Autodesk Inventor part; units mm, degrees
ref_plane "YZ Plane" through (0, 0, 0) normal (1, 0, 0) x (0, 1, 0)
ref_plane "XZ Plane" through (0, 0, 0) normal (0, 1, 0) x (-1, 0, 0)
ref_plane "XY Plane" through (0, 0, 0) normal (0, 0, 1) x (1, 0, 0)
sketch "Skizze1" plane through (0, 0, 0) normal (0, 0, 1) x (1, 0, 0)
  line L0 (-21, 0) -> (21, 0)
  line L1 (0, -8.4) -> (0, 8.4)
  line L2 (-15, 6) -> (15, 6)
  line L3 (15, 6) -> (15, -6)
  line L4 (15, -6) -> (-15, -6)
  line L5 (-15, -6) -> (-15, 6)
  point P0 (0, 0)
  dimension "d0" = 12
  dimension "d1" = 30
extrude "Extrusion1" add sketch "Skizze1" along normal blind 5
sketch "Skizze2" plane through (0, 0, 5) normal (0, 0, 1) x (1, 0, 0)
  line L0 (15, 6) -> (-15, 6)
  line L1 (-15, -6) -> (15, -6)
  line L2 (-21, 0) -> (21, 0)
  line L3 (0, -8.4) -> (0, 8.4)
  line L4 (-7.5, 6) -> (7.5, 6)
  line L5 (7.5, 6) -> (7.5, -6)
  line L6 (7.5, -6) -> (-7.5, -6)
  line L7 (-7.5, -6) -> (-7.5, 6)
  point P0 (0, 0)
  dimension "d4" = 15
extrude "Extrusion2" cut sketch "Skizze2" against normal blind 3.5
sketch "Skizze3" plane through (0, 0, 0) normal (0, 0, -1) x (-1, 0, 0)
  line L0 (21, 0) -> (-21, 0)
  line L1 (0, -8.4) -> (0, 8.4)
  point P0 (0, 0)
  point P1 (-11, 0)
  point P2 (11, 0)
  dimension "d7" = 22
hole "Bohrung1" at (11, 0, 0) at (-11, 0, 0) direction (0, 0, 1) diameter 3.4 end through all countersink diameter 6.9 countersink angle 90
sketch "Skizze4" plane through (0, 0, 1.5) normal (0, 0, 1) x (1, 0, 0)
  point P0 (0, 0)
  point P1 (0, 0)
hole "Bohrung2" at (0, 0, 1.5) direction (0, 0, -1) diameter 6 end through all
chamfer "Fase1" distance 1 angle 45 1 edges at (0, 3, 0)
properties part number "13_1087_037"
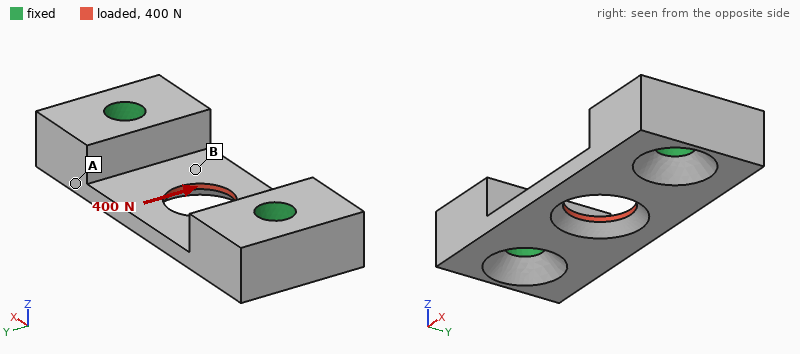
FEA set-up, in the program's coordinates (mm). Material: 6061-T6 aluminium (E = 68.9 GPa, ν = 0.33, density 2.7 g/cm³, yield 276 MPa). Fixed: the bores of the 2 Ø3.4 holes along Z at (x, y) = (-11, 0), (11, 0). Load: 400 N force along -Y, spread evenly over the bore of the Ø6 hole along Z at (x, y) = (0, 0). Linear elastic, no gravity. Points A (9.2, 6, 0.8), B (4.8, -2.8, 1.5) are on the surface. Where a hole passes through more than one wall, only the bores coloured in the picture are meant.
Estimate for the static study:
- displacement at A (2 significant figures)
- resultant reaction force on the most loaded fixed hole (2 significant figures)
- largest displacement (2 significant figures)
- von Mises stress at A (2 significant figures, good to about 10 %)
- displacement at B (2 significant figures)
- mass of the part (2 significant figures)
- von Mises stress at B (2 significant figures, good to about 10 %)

2.3 µm
200 N
8.6 µm
13 MPa
4.4 µm
2.7 g
31 MPa
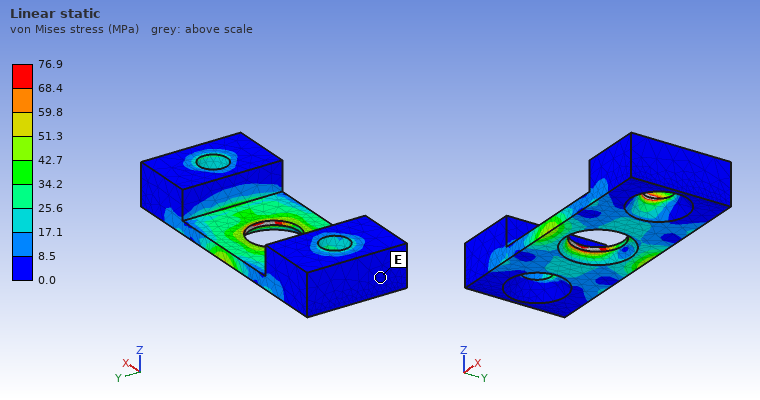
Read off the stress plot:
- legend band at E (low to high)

0.0 to 8.5 MPa
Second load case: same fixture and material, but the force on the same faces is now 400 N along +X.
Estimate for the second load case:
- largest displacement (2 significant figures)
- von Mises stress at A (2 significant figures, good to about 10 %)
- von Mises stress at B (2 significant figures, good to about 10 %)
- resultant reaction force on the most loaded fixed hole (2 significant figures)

3.4 µm
6.8 MPa
26 MPa
200 N
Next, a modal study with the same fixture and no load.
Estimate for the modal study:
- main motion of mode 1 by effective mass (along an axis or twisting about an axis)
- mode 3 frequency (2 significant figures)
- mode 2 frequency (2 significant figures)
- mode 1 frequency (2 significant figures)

along Z
53 kHz
32 kHz
27 kHz
